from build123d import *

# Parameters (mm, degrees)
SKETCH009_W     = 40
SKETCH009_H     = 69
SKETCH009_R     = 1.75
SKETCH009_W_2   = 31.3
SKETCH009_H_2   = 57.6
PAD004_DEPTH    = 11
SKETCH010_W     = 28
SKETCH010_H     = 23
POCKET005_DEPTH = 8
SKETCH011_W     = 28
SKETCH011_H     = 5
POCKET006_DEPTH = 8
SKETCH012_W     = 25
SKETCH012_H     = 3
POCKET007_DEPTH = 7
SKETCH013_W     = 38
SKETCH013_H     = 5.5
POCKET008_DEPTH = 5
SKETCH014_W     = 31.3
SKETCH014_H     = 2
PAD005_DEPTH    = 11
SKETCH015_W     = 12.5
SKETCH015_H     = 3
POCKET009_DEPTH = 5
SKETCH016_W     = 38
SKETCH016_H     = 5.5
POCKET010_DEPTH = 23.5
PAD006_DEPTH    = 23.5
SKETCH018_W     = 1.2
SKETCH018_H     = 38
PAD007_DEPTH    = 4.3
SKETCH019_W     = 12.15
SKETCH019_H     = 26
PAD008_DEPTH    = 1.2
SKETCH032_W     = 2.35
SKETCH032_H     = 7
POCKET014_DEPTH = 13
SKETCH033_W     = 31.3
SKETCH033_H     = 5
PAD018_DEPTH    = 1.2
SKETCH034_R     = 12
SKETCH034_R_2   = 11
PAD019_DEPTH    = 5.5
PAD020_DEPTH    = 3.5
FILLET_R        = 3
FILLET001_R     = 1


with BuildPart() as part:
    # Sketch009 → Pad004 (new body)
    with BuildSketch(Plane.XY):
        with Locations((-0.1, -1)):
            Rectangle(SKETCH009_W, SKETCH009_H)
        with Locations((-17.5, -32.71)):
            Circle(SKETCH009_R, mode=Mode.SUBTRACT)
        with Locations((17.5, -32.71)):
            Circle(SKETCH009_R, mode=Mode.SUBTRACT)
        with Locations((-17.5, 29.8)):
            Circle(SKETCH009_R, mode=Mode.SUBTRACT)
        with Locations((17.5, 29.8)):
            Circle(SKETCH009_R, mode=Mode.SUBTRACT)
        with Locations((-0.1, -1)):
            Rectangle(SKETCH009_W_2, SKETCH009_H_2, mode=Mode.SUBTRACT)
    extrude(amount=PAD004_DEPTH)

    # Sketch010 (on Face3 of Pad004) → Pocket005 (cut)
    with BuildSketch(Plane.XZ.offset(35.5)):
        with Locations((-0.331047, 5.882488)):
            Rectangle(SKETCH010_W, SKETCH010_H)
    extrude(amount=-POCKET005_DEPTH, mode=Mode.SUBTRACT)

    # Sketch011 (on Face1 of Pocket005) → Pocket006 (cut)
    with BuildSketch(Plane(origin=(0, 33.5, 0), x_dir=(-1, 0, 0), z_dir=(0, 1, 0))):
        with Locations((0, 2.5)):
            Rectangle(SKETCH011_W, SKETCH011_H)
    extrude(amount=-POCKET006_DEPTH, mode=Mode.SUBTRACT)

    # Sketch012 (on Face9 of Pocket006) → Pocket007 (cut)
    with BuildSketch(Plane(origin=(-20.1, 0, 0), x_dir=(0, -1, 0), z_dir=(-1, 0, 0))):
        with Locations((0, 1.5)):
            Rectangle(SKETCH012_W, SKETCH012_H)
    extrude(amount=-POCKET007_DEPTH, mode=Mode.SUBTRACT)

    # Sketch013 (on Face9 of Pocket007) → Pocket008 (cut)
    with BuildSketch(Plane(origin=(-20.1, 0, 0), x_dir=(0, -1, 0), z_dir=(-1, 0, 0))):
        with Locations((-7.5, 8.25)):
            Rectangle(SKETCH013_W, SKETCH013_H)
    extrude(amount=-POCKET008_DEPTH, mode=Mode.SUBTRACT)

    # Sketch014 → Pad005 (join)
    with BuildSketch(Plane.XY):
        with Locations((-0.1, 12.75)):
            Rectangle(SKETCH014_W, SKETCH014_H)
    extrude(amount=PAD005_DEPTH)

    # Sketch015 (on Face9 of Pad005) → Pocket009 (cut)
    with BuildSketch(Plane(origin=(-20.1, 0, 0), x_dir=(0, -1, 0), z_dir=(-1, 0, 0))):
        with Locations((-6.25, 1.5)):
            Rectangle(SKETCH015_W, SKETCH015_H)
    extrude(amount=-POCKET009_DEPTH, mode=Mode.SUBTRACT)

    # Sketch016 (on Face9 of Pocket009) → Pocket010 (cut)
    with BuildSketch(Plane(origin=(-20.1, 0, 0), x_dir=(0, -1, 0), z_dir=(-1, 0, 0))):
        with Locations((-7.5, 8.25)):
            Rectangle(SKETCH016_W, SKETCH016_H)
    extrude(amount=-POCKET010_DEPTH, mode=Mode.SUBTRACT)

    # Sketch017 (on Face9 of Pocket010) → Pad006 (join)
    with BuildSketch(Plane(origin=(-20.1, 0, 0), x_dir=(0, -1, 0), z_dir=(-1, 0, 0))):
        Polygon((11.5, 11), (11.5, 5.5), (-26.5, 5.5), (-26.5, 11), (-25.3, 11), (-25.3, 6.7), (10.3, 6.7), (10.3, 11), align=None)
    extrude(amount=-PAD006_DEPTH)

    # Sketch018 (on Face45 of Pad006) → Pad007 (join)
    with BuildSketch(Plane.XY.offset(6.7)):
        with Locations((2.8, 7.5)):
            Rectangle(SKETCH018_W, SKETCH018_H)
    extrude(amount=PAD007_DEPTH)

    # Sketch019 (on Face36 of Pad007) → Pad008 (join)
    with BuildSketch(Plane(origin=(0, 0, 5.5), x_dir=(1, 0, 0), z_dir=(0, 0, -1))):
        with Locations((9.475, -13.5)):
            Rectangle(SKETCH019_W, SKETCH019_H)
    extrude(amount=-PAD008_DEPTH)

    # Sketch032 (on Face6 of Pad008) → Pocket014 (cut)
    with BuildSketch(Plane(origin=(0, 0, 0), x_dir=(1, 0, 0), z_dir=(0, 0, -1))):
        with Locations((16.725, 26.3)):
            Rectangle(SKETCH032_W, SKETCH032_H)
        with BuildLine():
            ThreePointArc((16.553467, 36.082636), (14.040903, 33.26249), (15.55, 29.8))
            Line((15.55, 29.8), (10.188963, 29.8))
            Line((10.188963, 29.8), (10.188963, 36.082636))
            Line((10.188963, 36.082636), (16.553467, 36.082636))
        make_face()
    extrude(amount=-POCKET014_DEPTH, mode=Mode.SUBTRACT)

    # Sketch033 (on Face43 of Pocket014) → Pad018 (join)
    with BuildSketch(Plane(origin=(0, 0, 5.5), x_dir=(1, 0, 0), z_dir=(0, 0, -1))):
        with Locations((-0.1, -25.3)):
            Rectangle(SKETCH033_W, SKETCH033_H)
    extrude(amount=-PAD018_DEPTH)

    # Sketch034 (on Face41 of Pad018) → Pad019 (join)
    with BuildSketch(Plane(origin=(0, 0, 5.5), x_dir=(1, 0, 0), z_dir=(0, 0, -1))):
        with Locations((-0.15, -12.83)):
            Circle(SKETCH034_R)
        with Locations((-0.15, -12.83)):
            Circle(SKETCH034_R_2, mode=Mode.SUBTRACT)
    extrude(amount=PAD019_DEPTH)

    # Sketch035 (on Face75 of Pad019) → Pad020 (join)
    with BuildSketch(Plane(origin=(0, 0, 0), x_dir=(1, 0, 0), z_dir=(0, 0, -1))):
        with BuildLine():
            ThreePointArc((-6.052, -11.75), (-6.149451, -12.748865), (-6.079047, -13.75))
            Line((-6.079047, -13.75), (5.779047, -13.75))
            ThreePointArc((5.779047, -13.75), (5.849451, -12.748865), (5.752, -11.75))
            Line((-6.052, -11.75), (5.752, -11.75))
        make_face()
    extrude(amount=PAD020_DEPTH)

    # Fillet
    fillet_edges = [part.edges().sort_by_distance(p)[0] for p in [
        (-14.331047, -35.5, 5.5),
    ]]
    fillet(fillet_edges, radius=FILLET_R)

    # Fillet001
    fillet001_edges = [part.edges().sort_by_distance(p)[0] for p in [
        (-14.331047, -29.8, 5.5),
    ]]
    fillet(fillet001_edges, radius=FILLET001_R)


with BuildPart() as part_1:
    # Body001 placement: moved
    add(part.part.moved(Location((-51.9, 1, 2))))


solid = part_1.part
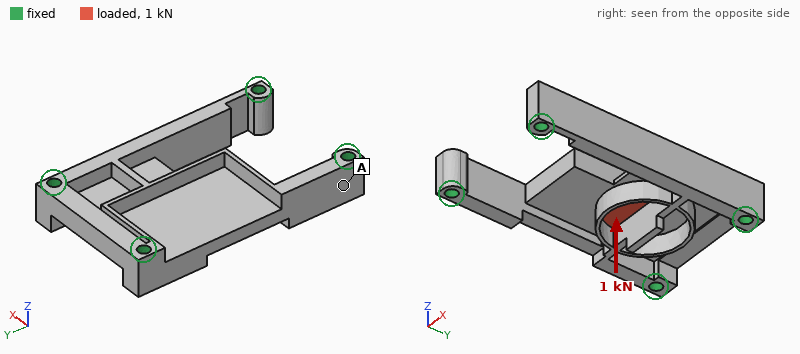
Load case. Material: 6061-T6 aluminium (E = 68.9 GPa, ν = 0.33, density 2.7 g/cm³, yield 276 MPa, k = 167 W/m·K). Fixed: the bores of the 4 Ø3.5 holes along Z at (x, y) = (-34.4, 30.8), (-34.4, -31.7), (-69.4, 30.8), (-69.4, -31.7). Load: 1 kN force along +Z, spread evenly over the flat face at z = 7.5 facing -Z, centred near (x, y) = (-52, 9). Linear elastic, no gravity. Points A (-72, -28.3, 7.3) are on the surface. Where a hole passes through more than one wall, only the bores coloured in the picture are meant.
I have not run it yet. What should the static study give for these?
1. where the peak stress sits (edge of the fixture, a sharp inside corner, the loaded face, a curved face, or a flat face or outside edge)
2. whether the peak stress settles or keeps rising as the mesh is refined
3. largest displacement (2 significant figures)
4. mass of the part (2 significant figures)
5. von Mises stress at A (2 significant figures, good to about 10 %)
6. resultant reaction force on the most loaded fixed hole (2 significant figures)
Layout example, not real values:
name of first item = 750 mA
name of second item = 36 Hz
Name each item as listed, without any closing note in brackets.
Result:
where the peak stress sits = a sharp inside corner
whether the peak stress settles or keeps rising as the mesh is refined = keeps rising
largest displacement = 0.18 mm
mass of the part = 24 g
von Mises stress at A = 20 MPa
resultant reaction force on the most loaded fixed hole = 390 N
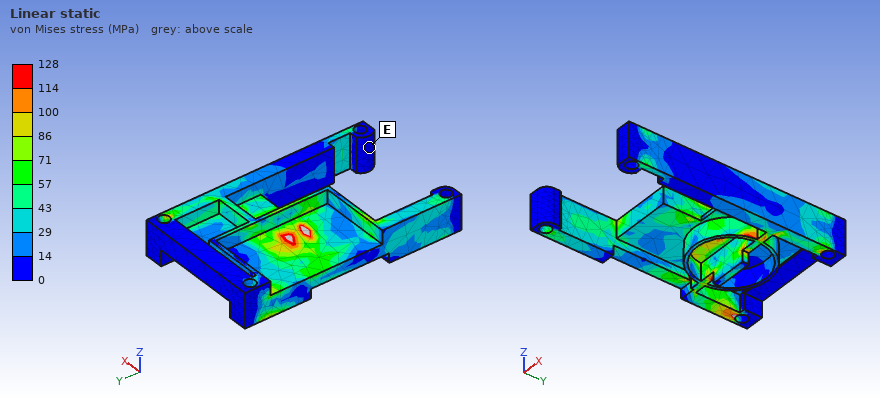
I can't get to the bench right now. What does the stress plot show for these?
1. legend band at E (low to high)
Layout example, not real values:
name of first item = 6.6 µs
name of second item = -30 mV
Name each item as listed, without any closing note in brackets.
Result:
legend band at E = 0 to 14 MPa
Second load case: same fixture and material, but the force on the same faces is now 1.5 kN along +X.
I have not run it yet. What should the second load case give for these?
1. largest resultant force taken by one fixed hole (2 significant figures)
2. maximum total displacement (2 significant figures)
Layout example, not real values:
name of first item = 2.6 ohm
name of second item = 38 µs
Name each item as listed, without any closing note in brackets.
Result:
largest resultant force taken by one fixed hole = 990 N
maximum total displacement = 33 µm
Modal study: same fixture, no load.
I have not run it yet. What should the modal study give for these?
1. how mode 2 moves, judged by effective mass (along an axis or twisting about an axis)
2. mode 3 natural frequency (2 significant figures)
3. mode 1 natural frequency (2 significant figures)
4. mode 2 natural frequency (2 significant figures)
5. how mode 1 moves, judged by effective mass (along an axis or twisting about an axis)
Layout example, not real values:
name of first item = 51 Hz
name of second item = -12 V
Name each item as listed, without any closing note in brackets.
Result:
how mode 2 moves, judged by effective mass = along X
mode 3 natural frequency = 11 kHz
mode 1 natural frequency = 6500 Hz
mode 2 natural frequency = 10000 Hz
how mode 1 moves, judged by effective mass = along Z
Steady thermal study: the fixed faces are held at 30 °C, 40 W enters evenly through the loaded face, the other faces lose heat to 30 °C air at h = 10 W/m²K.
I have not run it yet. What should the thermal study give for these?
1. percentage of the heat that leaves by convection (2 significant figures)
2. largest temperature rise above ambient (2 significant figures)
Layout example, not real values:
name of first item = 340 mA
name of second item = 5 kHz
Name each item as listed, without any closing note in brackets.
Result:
percentage of the heat that leaves by convection = 3.8 %
largest temperature rise above ambient = 55 K
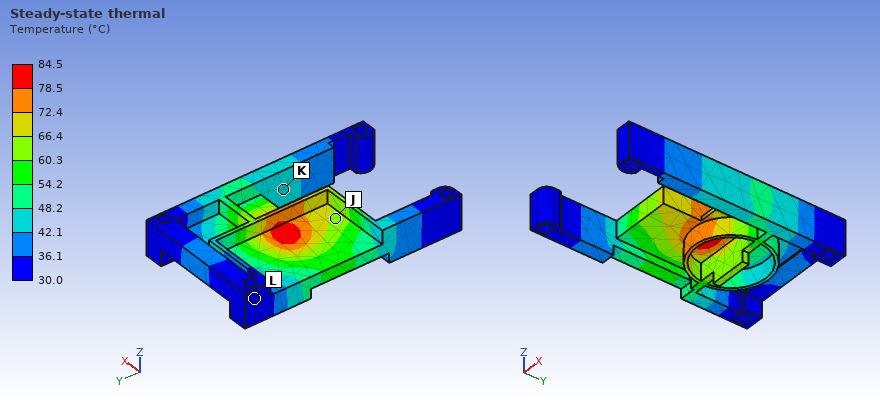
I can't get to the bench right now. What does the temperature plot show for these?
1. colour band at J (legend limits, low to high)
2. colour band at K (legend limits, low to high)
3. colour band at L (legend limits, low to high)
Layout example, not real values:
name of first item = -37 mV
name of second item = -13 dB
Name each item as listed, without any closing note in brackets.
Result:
colour band at J = 60.3 to 66.4 °C
colour band at K = 42.1 to 48.2 °C
colour band at L = 30.0 to 36.1 °C
